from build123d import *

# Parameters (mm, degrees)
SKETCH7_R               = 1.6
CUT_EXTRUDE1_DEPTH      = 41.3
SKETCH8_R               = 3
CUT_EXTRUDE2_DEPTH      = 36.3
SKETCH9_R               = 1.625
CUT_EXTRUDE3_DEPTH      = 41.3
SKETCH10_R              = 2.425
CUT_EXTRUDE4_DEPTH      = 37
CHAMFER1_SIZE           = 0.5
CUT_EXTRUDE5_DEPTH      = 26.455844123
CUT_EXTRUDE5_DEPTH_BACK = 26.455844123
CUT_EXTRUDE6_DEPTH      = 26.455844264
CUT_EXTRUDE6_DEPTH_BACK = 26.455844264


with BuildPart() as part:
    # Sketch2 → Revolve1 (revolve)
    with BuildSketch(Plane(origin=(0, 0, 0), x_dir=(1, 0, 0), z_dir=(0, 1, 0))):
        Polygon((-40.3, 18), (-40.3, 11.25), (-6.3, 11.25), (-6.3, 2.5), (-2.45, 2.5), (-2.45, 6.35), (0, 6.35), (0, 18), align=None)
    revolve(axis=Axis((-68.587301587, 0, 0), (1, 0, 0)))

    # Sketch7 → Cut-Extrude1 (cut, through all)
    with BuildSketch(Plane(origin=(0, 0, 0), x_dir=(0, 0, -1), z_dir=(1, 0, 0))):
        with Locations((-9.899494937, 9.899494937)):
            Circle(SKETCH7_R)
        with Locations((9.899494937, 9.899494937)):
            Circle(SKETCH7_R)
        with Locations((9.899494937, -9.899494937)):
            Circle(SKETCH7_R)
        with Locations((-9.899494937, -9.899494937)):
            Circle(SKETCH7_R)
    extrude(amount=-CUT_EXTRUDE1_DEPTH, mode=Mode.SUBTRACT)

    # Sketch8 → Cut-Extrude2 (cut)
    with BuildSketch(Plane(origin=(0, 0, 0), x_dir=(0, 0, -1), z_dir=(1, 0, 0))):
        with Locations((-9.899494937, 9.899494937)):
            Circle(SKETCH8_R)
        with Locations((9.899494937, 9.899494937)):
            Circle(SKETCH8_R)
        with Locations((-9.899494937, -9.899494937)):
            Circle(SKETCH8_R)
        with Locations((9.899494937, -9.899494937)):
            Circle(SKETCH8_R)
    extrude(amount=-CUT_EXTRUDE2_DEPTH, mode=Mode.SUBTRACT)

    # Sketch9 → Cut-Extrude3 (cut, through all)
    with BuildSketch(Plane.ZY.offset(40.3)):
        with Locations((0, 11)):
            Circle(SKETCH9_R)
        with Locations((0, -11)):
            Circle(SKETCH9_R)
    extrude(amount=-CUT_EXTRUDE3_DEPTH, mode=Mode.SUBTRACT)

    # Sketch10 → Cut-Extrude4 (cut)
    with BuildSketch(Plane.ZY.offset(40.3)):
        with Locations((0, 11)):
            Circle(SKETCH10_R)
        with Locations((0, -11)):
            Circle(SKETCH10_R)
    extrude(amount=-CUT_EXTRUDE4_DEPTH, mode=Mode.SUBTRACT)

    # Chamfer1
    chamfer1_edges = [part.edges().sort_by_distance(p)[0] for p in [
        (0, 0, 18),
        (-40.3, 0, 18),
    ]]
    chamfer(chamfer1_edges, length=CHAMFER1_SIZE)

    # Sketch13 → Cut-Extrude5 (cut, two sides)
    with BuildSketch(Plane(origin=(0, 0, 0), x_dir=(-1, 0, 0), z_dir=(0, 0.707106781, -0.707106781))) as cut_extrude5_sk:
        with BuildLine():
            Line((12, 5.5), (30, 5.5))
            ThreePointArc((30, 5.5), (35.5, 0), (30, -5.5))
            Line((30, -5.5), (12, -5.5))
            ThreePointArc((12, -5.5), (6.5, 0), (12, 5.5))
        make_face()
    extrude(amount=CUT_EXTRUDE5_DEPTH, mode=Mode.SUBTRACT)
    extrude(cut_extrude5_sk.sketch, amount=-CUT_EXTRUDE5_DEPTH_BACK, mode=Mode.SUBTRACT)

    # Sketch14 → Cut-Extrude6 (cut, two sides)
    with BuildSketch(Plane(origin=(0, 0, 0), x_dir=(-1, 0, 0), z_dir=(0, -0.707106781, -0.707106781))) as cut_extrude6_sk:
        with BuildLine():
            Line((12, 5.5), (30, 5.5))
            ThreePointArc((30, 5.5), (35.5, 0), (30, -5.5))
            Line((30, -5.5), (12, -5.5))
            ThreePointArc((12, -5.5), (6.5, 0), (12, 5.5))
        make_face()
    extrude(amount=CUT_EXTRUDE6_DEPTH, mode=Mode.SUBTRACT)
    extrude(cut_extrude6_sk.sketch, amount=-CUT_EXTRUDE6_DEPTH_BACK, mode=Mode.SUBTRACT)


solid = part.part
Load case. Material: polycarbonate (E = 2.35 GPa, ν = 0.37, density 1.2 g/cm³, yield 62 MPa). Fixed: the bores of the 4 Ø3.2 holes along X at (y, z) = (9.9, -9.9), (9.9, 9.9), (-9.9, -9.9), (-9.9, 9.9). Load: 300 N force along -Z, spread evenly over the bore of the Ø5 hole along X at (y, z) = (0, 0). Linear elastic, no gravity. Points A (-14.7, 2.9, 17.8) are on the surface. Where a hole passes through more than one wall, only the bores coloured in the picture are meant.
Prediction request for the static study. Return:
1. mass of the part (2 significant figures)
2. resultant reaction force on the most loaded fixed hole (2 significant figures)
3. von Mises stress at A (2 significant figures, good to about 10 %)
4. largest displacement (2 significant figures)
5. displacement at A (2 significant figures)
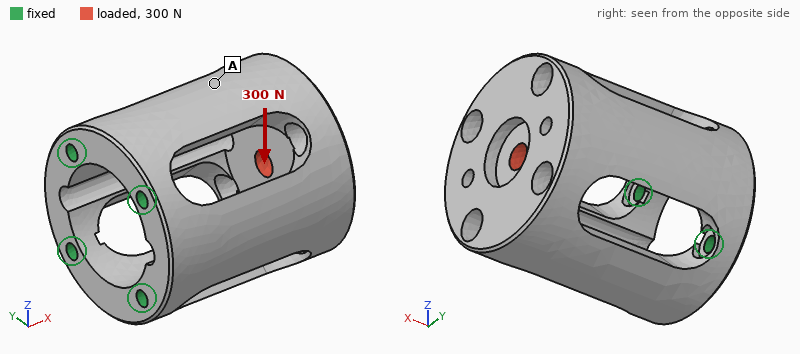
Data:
21 g
240 N
2.6 MPa
0.47 mm
0.37 mm
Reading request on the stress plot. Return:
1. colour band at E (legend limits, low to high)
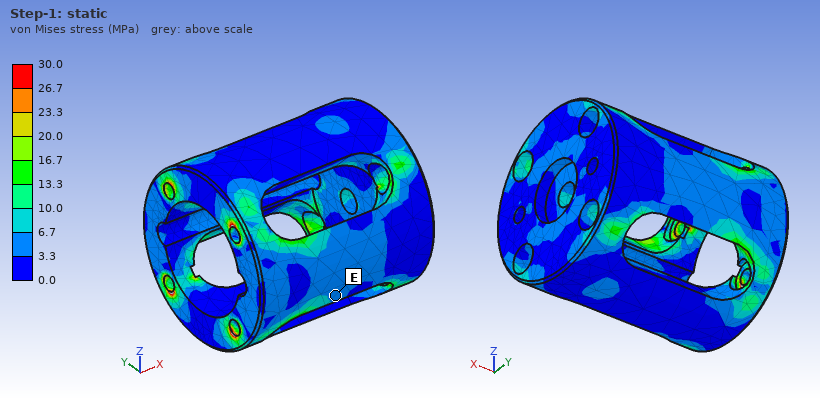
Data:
3.3 to 6.7 MPa
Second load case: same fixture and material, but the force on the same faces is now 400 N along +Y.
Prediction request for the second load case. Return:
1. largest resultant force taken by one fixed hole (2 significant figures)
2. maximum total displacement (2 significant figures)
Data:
320 N
0.63 mm
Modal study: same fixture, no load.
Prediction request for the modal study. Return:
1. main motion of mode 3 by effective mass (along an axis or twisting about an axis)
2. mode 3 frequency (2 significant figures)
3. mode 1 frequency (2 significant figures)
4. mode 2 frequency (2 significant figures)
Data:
twisting about X
2600 Hz
1300 Hz
1300 Hz
